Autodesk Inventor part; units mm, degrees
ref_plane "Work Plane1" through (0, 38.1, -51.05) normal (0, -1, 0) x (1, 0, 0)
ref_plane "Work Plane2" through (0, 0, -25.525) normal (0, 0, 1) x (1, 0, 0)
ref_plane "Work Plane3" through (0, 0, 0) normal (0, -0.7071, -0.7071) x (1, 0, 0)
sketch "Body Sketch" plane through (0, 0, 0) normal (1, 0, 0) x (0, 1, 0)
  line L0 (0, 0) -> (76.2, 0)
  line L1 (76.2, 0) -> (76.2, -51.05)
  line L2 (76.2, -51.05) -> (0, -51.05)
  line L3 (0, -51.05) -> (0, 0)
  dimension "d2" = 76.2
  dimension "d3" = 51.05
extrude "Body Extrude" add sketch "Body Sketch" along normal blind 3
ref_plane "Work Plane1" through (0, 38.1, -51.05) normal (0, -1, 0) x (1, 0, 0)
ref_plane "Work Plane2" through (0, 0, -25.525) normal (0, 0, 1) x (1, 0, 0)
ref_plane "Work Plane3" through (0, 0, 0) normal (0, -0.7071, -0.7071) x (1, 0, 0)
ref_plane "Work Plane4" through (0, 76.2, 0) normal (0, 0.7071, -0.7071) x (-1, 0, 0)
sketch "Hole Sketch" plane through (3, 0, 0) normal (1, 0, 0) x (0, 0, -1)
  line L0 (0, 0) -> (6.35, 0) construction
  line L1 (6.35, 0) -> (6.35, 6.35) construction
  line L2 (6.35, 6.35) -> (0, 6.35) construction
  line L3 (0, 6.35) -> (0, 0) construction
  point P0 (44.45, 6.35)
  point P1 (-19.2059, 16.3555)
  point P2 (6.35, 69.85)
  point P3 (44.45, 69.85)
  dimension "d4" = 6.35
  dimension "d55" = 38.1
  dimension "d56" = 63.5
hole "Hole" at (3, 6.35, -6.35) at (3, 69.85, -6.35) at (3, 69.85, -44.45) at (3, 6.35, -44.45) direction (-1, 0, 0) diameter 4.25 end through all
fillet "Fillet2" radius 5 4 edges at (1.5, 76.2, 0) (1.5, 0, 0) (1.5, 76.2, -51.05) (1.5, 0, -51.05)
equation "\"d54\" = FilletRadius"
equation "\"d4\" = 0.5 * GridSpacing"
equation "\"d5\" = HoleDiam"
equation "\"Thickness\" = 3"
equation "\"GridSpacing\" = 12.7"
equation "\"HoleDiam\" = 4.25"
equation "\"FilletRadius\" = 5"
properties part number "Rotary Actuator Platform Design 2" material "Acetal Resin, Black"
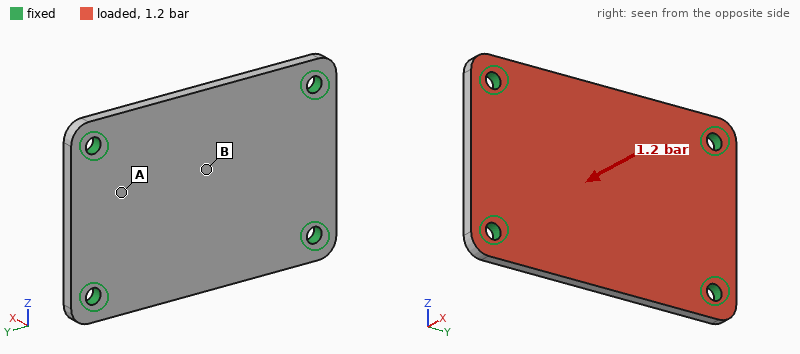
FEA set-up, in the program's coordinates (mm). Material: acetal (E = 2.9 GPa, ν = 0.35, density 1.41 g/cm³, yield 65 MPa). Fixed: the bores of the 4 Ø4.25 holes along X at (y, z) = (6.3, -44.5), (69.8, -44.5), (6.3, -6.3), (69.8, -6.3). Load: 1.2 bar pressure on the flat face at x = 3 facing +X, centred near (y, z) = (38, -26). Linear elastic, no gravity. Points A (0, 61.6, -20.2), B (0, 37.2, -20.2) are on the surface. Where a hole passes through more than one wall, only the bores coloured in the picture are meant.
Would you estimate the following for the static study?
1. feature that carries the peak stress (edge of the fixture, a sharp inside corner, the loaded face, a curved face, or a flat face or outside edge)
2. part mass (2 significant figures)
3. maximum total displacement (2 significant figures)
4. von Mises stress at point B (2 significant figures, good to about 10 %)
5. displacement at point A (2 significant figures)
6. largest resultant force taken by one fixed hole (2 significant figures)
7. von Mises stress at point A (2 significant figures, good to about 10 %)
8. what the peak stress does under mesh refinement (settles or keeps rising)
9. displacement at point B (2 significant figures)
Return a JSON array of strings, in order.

["edge of the fixture", "16 g", "0.91 mm", "12 MPa", "0.34 mm", "120 N", "6.4 MPa", "keeps rising", "0.91 mm"]
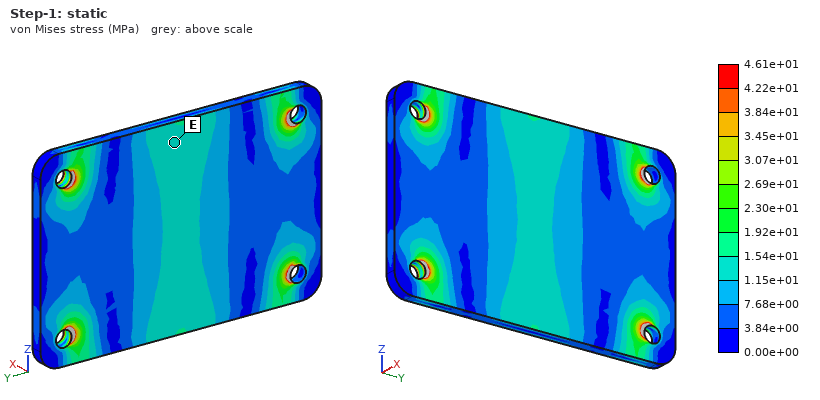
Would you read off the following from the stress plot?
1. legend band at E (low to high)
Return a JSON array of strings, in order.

["1.15e+01 to 1.54e+01 MPa"]
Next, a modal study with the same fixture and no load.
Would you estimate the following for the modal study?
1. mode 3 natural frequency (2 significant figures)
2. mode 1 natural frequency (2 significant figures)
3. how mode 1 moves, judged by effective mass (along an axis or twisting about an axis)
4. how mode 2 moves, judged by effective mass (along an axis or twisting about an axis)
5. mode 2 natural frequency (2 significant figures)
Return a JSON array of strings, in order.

["2500 Hz", "1000 Hz", "along X", "twisting about Y", "1500 Hz"]
